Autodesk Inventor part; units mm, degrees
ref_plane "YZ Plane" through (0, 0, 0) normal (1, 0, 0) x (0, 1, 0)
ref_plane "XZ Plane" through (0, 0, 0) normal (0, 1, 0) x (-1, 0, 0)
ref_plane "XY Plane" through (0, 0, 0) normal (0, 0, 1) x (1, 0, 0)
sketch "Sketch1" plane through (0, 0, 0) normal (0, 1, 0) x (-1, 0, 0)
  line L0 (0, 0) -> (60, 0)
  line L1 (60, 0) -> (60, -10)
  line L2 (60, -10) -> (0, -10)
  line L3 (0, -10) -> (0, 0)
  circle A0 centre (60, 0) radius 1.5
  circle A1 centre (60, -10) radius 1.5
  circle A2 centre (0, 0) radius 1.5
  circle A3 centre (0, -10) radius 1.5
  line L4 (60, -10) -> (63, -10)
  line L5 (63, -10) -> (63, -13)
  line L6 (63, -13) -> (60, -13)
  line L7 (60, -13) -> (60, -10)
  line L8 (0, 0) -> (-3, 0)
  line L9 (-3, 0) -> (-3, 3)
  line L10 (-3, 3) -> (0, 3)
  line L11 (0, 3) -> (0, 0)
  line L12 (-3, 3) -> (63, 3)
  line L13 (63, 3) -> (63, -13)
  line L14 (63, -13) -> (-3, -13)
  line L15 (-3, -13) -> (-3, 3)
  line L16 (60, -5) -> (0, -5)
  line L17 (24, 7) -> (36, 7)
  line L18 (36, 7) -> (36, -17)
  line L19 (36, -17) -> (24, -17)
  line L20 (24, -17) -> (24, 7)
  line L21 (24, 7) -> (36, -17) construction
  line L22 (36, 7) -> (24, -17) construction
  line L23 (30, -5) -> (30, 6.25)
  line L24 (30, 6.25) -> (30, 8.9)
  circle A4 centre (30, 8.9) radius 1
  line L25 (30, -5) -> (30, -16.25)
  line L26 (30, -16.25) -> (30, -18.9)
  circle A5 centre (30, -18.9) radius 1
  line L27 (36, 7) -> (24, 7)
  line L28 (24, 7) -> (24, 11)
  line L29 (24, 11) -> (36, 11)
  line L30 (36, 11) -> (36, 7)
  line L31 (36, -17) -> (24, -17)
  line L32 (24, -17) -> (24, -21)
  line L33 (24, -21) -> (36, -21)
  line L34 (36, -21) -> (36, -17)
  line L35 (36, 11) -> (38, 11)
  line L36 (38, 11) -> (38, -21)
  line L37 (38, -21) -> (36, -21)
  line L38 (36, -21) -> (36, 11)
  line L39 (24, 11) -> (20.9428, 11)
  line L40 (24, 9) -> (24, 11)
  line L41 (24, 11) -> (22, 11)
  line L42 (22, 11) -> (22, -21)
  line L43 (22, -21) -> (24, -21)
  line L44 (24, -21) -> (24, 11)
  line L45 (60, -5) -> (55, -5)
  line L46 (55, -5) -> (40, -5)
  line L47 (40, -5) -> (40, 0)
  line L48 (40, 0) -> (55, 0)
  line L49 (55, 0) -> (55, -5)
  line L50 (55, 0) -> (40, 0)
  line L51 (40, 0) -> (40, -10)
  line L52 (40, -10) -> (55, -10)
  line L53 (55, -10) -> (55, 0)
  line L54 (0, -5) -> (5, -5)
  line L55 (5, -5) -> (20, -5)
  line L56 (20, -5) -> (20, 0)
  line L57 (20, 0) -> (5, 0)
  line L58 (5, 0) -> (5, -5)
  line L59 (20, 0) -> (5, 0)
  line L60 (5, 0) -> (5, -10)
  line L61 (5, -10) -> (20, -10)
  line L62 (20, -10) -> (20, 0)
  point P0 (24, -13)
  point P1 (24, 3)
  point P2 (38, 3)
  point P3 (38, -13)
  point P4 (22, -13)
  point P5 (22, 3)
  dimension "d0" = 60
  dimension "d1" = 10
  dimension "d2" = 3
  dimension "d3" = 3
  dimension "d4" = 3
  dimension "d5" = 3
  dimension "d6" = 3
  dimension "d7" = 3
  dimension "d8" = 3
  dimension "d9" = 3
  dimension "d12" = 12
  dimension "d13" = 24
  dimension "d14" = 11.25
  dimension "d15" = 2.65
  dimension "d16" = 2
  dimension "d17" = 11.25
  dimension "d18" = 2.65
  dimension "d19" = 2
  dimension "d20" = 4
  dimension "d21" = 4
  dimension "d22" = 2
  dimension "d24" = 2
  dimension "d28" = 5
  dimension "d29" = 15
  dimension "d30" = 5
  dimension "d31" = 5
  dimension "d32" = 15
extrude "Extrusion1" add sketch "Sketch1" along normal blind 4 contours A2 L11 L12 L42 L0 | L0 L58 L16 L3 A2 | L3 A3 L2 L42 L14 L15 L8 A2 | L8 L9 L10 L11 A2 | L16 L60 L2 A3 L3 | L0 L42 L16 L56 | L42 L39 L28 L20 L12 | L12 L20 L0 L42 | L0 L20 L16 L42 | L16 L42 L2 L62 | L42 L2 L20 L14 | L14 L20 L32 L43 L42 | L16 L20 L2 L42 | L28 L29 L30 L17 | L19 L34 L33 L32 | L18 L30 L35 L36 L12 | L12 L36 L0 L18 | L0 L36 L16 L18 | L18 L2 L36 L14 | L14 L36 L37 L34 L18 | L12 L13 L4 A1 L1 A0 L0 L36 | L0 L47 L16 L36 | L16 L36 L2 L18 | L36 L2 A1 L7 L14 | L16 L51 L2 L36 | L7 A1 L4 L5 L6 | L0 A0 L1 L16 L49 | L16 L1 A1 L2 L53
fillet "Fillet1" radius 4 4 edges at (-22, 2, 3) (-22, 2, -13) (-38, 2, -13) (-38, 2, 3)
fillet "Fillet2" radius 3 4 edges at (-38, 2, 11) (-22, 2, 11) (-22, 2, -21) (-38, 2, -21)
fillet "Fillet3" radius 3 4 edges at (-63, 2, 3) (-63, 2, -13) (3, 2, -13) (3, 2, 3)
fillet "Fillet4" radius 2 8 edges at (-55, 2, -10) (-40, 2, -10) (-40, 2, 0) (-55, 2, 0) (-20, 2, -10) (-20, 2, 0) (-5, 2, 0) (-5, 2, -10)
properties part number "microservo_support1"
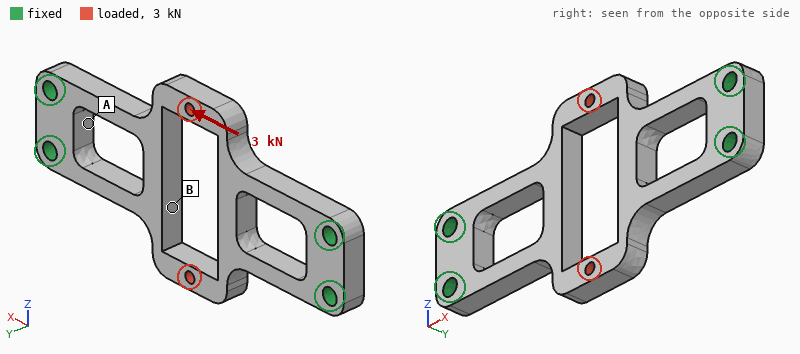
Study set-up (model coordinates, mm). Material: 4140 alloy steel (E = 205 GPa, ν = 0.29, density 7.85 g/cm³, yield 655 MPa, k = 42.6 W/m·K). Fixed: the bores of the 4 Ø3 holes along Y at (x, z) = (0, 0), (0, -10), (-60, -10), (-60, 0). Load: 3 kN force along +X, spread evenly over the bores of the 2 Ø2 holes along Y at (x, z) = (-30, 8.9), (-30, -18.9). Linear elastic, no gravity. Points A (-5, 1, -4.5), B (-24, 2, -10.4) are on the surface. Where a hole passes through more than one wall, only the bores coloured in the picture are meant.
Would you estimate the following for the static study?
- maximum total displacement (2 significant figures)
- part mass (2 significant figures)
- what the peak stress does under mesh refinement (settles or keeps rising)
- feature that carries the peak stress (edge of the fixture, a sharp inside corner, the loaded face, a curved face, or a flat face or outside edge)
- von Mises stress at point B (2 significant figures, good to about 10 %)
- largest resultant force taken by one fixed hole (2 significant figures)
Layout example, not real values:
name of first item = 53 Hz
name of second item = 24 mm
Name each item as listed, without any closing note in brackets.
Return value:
maximum total displacement = 31 µm
part mass = 22 g
what the peak stress does under mesh refinement = keeps rising
feature that carries the peak stress = a sharp inside corner
von Mises stress at point B = 120 MPa
largest resultant force taken by one fixed hole = 750 N
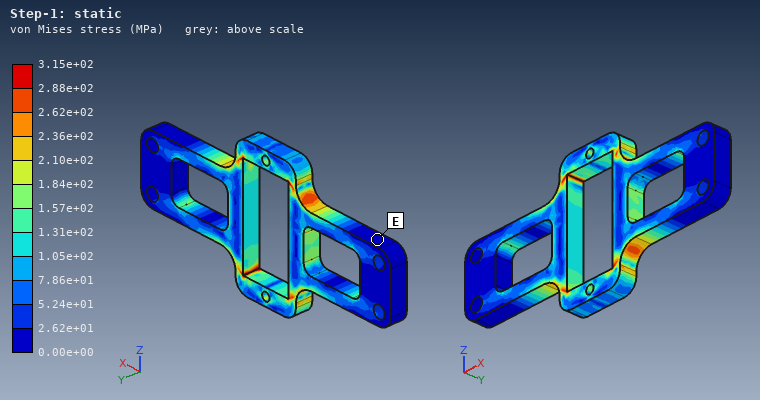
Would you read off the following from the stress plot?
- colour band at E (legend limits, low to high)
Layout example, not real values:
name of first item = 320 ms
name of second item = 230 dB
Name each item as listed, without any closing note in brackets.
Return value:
colour band at E = 0.00e+00 to 2.62e+01 MPa
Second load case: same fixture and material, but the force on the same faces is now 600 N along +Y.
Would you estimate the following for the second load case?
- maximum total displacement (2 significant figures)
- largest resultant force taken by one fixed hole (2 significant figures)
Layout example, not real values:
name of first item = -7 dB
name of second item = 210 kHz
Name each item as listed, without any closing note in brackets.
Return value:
maximum total displacement = 0.13 mm
largest resultant force taken by one fixed hole = 150 N
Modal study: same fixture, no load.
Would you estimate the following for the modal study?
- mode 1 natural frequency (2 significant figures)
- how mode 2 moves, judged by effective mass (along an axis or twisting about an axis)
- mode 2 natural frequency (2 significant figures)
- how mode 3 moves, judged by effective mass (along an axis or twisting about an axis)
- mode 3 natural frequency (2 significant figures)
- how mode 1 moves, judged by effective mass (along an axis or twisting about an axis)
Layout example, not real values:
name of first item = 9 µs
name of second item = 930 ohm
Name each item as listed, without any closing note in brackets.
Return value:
mode 1 natural frequency = 4100 Hz
how mode 2 moves, judged by effective mass = twisting about X
mode 2 natural frequency = 4700 Hz
how mode 3 moves, judged by effective mass = along Z
mode 3 natural frequency = 6400 Hz
how mode 1 moves, judged by effective mass = along Y
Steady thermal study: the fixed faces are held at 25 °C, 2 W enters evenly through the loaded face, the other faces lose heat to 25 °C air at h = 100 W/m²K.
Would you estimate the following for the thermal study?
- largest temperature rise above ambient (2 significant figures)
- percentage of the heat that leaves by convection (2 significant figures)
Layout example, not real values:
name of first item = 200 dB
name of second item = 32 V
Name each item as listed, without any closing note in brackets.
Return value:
largest temperature rise above ambient = 15 K
percentage of the heat that leaves by convection = 69 %
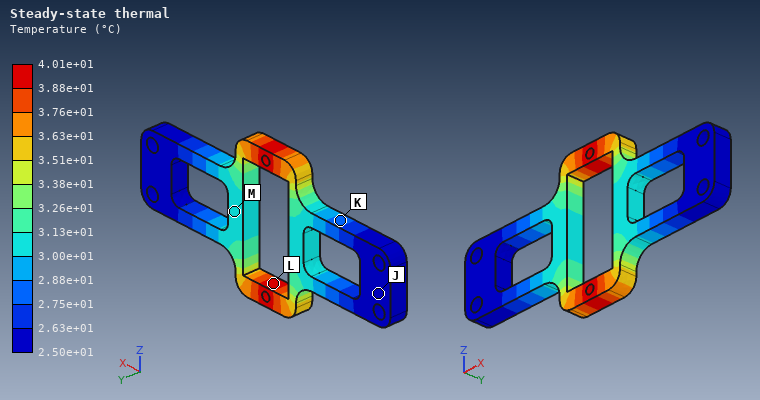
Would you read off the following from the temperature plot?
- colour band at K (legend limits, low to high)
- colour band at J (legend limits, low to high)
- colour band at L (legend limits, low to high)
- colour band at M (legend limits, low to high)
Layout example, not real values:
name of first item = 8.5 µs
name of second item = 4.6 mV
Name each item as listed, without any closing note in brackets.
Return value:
colour band at K = 2.75e+01 to 2.88e+01 °C
colour band at J = 2.50e+01 to 2.63e+01 °C
colour band at L = 3.88e+01 to 4.01e+01 °C
colour band at M = 3.00e+01 to 3.13e+01 °C
